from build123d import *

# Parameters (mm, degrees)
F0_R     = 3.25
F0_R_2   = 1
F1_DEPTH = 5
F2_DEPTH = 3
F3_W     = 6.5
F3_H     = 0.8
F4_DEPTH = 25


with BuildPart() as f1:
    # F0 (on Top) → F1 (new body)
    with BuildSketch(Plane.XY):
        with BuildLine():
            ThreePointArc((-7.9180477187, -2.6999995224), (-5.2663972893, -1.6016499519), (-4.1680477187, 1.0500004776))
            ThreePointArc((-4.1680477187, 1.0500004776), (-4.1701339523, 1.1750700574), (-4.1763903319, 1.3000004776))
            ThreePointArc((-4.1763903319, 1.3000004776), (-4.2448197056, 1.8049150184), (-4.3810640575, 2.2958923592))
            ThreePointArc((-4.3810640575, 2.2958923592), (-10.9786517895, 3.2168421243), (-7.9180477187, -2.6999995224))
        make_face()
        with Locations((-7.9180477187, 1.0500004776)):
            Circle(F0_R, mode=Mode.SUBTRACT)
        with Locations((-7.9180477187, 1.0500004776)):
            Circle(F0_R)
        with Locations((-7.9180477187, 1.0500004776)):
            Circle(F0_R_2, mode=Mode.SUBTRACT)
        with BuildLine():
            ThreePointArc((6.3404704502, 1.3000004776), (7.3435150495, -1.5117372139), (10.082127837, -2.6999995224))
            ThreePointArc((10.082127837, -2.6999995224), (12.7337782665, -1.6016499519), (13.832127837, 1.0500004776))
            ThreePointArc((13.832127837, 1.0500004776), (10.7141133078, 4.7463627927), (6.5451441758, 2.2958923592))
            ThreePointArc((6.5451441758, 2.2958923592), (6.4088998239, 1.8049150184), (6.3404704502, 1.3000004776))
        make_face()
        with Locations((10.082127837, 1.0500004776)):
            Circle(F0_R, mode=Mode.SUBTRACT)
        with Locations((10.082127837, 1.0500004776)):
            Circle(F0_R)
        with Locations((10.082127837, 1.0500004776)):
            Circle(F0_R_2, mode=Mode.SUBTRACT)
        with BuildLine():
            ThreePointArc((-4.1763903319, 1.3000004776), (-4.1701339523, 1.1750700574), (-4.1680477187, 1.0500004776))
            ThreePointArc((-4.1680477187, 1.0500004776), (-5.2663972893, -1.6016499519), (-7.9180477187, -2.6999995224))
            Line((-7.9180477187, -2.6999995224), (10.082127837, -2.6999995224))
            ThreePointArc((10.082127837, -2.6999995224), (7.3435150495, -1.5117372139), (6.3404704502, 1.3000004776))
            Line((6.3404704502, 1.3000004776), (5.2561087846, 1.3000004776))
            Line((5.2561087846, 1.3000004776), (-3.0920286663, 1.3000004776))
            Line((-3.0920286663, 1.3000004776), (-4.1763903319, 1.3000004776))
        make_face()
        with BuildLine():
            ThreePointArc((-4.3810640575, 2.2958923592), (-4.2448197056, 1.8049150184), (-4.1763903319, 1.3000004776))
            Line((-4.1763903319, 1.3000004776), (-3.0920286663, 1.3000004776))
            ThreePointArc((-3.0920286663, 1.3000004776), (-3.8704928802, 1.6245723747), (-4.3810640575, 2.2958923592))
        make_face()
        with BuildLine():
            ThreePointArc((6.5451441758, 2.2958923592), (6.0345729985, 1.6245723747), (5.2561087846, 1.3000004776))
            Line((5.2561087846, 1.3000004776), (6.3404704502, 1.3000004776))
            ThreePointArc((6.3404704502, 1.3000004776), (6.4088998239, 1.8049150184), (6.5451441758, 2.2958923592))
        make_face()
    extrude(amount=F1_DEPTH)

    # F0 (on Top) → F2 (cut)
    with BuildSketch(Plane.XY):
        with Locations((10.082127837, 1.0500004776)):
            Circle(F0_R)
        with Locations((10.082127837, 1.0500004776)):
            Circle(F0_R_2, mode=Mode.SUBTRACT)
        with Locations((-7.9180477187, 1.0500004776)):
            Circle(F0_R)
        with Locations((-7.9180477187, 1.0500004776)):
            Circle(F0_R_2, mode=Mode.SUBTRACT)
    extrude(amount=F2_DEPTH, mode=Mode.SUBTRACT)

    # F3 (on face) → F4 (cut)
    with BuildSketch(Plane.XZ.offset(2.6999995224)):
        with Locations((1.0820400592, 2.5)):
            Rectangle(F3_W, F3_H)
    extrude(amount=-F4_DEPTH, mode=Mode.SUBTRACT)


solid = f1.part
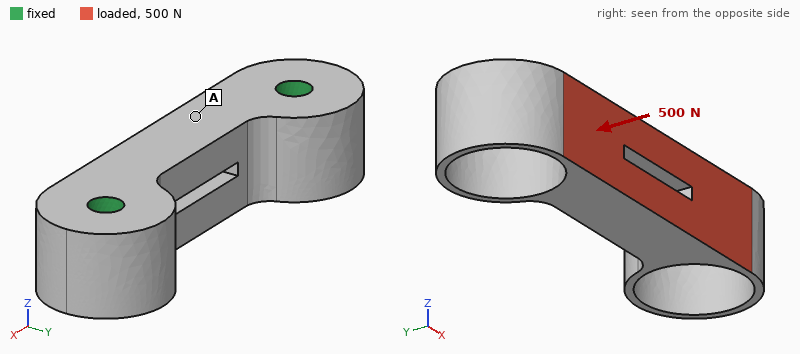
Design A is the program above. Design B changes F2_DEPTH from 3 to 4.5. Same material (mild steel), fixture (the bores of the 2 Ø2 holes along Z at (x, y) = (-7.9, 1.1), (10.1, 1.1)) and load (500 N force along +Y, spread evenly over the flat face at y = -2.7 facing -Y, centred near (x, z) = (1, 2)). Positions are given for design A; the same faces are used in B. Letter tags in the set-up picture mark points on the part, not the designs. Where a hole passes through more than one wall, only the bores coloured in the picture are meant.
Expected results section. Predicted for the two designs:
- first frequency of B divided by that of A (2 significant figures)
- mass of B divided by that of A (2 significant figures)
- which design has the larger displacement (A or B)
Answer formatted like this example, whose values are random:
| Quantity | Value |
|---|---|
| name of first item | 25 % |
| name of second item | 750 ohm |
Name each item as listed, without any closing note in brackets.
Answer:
| Quantity | Value |
|---|---|
| first frequency of B divided by that of A | 0.26 |
| mass of B divided by that of A | 0.80 |
| which design has the larger displacement | B |
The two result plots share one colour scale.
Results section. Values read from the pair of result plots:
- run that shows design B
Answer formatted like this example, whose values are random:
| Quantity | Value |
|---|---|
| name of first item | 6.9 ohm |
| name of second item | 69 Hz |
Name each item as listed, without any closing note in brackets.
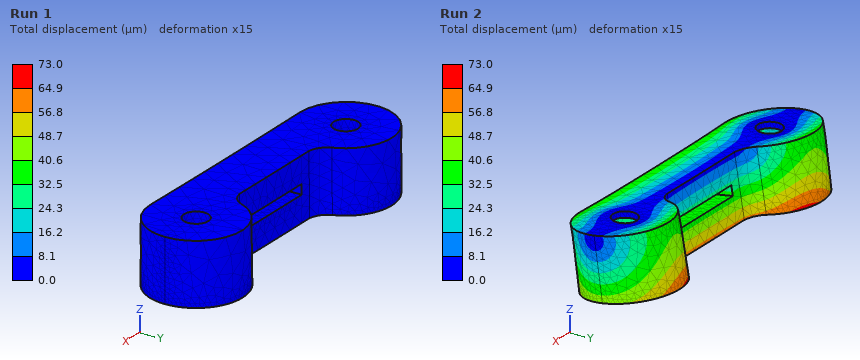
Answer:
| Quantity | Value |
|---|---|
| run that shows design B | Run 2 |
